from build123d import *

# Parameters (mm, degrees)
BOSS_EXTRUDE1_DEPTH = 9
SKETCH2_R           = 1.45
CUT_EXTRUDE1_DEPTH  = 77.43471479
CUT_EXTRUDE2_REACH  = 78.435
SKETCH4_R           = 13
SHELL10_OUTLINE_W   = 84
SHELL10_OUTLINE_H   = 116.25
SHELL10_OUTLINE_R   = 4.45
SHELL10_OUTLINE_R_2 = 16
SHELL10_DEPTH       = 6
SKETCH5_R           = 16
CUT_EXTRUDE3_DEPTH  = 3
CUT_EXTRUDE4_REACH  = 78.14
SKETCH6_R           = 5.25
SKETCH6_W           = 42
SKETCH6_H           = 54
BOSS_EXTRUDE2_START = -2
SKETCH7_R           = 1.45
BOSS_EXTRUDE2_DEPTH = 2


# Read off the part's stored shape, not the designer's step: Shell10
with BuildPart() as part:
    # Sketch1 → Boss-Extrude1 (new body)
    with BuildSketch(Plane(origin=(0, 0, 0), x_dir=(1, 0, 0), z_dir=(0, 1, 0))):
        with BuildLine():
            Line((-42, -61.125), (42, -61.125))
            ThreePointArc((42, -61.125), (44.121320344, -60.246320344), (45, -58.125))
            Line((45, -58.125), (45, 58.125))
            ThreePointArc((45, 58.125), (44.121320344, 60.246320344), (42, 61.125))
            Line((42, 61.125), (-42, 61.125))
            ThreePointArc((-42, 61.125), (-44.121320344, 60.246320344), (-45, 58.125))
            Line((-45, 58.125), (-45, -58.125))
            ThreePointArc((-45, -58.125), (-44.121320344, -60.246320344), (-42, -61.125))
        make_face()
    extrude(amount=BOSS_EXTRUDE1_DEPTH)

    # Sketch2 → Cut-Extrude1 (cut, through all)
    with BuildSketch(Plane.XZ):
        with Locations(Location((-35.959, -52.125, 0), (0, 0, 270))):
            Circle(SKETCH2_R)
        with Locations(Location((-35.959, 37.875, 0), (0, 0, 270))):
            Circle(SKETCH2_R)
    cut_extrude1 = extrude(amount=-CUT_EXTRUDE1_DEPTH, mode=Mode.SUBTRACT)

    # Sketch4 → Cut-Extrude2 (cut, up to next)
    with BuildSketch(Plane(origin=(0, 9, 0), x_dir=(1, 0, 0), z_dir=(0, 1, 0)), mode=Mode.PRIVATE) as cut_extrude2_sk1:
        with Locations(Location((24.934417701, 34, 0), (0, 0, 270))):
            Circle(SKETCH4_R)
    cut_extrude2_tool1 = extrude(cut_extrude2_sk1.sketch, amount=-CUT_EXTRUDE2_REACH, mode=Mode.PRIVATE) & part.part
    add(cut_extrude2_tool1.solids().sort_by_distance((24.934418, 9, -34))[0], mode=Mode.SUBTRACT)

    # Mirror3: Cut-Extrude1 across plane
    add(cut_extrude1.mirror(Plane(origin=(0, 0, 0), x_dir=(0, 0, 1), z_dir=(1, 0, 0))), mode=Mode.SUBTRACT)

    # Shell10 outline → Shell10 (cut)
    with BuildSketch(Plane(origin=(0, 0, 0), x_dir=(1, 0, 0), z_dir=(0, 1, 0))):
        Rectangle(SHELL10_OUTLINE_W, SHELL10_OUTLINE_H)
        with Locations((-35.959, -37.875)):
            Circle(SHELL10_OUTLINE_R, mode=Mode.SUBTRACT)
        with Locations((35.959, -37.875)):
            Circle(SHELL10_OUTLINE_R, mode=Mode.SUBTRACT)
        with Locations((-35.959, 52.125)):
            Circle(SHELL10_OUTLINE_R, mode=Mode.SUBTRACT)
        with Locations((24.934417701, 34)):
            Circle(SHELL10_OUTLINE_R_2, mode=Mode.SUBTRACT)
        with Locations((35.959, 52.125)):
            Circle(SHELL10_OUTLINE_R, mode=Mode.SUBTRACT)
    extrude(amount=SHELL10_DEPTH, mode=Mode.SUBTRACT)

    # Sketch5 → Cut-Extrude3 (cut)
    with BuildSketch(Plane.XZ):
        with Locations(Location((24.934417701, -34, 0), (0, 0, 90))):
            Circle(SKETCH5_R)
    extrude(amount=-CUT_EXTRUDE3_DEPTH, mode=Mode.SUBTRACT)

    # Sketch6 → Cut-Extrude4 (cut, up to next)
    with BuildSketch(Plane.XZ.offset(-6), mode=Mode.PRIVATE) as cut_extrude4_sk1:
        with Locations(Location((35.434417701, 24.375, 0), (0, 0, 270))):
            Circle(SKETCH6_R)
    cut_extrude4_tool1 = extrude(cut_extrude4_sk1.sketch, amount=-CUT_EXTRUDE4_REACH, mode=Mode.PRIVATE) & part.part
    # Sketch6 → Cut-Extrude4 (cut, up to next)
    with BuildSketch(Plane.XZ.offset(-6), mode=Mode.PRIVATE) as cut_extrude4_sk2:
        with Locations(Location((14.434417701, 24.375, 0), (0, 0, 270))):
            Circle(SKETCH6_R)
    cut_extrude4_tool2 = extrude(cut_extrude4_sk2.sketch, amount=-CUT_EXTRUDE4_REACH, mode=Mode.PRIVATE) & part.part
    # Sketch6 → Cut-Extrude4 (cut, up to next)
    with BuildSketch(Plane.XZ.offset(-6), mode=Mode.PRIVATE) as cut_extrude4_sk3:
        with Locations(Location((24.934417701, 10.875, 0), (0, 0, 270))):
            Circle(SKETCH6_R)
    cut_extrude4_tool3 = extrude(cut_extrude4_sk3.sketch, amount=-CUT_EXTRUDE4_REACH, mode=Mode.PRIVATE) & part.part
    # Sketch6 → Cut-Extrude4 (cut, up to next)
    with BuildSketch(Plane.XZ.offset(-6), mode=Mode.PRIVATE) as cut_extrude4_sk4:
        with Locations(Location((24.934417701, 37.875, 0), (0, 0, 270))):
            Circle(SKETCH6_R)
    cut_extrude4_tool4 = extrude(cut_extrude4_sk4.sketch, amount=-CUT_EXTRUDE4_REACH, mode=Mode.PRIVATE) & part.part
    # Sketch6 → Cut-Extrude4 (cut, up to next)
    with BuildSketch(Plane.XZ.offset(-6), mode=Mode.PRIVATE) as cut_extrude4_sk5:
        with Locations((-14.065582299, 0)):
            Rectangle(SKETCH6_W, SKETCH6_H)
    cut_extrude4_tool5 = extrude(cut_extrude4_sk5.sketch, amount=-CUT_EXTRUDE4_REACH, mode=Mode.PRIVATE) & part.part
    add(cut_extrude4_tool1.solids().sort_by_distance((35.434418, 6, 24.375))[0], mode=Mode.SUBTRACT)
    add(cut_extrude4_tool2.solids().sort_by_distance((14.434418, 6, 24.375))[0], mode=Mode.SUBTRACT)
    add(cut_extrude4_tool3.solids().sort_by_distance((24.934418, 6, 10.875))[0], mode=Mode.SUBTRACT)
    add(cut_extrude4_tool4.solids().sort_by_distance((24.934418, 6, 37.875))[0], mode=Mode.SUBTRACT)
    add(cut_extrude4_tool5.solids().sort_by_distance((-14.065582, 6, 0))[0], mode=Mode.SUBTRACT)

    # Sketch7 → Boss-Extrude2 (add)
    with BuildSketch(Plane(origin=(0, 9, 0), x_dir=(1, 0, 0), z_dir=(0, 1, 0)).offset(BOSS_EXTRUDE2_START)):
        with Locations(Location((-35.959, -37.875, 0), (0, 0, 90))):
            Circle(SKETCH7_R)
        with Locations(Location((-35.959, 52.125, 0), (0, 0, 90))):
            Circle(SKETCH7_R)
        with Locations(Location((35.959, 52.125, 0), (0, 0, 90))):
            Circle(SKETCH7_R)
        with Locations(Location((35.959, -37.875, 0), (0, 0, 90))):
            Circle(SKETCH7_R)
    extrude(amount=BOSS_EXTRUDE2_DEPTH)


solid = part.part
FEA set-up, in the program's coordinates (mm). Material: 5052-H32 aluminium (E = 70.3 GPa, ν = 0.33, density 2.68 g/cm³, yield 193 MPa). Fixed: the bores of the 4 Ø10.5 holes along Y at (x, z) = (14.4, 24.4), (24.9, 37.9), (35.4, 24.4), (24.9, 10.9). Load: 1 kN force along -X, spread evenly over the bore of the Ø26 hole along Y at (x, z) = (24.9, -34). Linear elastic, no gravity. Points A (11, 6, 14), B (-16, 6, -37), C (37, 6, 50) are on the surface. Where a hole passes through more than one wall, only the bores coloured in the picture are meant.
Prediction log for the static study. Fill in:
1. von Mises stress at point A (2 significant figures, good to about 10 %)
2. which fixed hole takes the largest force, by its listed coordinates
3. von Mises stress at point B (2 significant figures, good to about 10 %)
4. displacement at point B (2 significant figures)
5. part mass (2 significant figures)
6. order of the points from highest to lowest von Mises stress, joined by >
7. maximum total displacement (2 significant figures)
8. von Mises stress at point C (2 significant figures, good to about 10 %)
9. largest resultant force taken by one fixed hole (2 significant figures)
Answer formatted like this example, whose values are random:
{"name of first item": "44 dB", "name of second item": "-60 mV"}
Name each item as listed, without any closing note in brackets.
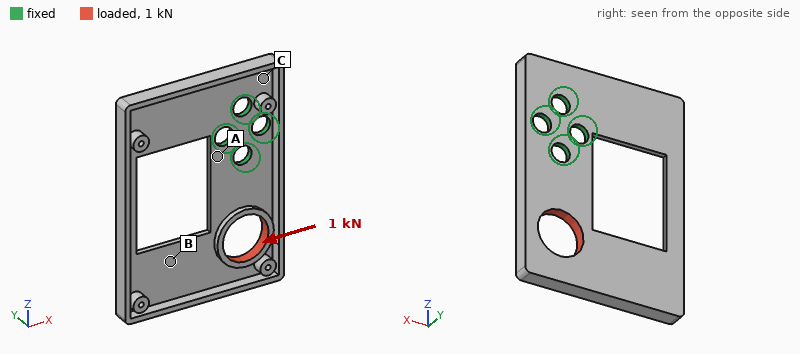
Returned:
{"von Mises stress at point A": "21 MPa", "which fixed hole takes the largest force, by its listed coordinates": "(24.9, 10.9)", "von Mises stress at point B": "10 MPa", "displacement at point B": "0.099 mm", "part mass": "89 g", "order of the points from highest to lowest von Mises stress, joined by >": "A > B > C", "maximum total displacement": "0.21 mm", "von Mises stress at point C": "4.8 MPa", "largest resultant force taken by one fixed hole": "1.3 kN"}
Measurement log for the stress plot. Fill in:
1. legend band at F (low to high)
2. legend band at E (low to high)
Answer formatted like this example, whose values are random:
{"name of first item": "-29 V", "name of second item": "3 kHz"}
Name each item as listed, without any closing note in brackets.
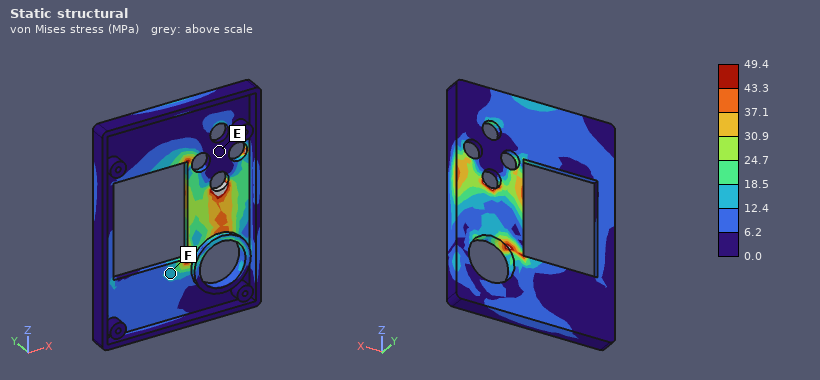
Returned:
{"legend band at F": "12.4 to 18.5 MPa", "legend band at E": "0.0 to 6.2 MPa"}
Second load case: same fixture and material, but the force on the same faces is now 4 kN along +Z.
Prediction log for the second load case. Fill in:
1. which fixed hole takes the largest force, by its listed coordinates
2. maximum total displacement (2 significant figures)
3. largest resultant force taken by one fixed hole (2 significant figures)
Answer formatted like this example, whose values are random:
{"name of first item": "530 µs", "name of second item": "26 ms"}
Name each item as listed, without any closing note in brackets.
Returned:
{"which fixed hole takes the largest force, by its listed coordinates": "(24.9, 10.9)", "maximum total displacement": "0.44 mm", "largest resultant force taken by one fixed hole": "2.1 kN"}
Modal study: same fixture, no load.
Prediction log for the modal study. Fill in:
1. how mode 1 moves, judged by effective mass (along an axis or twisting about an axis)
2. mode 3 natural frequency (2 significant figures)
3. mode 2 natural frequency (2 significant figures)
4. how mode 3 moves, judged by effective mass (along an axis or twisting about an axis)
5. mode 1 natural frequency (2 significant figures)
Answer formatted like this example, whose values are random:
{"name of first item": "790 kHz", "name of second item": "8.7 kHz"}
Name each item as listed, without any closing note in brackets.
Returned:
{"how mode 1 moves, judged by effective mass": "along Y", "mode 3 natural frequency": "930 Hz", "mode 2 natural frequency": "680 Hz", "how mode 3 moves, judged by effective mass": "along Y", "mode 1 natural frequency": "320 Hz"}
